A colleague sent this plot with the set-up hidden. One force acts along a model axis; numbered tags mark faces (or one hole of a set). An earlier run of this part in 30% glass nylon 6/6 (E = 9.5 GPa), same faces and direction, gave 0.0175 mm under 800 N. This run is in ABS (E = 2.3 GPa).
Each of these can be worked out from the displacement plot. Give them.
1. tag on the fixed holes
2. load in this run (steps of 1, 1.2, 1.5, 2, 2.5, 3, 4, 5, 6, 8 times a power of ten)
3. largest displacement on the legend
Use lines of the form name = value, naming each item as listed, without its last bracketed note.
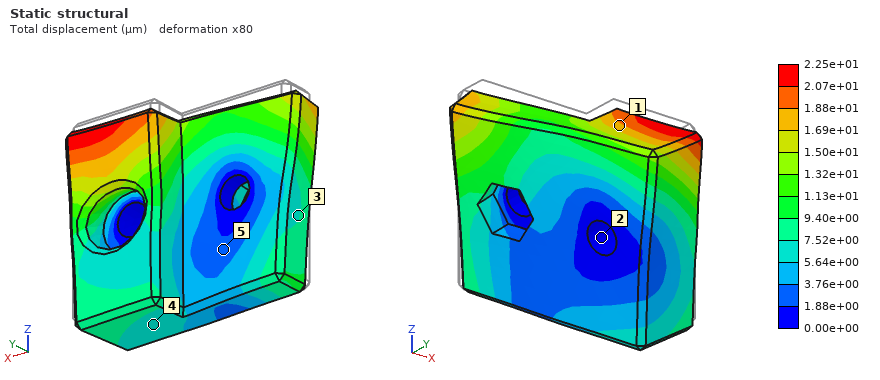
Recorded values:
tag on the fixed holes = 2
load in this run = 250 N
largest displacement on the legend = 2.25e+01 µm
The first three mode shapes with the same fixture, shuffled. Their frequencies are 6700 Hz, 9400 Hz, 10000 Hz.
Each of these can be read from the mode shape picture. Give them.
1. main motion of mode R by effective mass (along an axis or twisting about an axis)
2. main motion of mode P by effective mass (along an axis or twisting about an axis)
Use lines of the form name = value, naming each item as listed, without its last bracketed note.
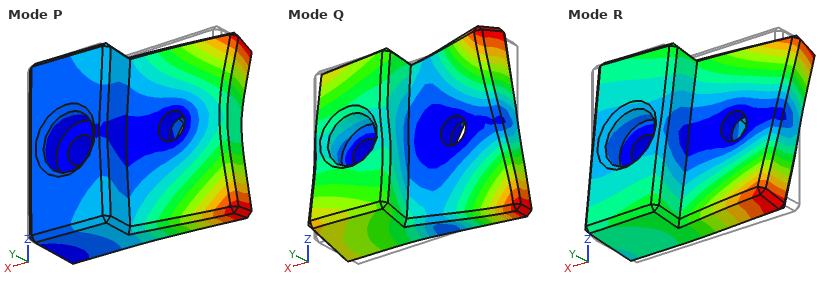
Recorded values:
main motion of mode R by effective mass = twisting about X
main motion of mode P by effective mass = along Y
